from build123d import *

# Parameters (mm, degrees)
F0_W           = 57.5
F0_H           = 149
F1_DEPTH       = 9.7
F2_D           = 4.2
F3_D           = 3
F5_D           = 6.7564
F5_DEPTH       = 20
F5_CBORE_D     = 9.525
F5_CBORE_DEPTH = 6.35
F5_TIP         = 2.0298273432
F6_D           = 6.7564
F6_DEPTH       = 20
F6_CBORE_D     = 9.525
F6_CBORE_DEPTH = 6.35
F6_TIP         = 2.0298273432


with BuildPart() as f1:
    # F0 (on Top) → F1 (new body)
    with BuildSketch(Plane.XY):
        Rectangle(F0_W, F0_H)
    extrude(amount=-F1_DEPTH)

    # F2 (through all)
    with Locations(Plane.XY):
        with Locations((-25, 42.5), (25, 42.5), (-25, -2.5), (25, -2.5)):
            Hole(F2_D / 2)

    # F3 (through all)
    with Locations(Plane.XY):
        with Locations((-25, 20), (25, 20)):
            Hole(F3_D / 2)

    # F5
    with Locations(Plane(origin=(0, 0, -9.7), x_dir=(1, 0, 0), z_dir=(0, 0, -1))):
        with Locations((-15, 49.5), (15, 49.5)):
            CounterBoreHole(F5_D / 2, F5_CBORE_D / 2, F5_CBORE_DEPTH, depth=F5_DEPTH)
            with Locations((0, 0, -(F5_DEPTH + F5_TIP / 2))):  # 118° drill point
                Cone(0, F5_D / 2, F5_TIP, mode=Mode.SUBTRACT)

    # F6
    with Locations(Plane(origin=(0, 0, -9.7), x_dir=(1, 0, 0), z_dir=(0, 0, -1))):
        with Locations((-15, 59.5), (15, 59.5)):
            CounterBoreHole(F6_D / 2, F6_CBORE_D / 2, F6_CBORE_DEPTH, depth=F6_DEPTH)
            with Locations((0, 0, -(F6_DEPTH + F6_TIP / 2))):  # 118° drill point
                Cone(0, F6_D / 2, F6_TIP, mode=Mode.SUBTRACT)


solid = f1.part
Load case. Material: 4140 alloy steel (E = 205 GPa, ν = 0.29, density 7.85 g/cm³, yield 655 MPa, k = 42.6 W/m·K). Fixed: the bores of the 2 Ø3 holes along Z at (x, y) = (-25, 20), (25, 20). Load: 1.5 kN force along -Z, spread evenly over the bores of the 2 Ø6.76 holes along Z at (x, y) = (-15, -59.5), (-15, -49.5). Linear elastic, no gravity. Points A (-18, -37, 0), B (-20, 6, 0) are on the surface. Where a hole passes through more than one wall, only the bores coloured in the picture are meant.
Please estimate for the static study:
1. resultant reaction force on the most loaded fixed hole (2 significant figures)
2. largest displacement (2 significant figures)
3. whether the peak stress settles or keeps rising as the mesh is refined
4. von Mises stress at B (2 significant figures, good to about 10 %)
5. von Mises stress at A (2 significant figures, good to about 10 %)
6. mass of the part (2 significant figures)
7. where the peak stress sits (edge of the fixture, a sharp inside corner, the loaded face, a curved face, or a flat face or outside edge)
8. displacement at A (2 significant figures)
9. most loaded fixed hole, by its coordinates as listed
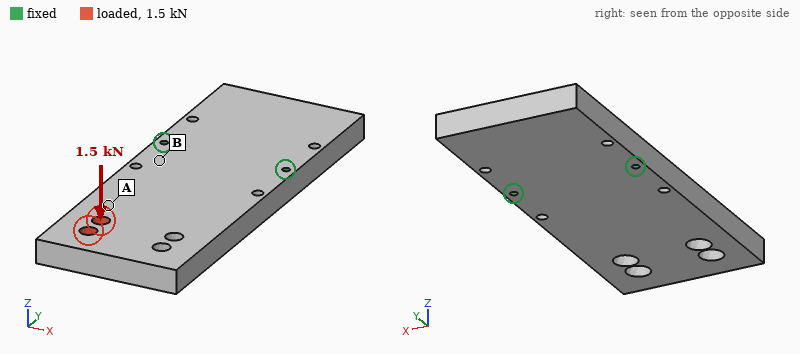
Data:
1.2 kN
0.47 mm
keeps rising
120 MPa
42 MPa
630 g
edge of the fixture
0.24 mm
(-25, 20)
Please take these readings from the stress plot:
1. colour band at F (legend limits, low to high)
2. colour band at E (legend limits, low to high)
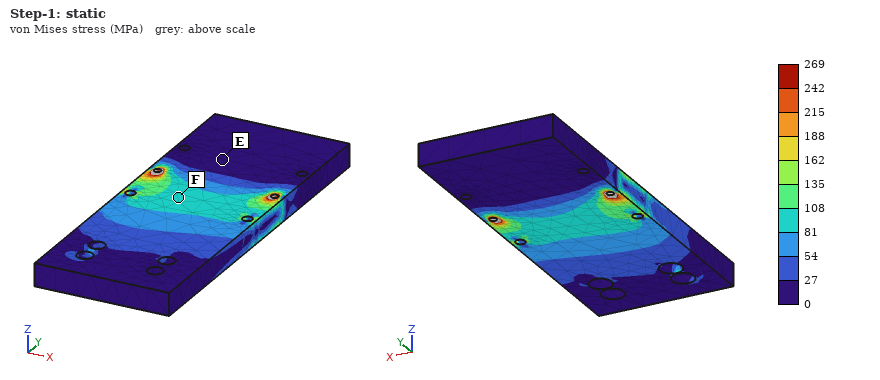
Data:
81 to 108 MPa
0 to 27 MPa
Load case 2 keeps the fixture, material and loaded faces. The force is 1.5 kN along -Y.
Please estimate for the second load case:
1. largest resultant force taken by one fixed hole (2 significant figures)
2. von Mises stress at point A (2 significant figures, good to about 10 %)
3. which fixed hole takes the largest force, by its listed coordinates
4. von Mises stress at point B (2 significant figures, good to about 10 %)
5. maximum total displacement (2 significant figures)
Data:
1.2 kN
12 MPa
(-25, 20)
12 MPa
30 µm
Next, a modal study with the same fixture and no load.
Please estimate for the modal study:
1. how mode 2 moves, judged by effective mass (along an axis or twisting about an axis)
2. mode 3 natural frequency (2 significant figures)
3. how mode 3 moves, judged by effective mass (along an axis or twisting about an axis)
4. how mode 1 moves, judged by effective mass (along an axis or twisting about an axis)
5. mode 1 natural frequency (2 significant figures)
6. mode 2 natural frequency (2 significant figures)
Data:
along Z
3000 Hz
twisting about Y
along Z
780 Hz
2200 Hz
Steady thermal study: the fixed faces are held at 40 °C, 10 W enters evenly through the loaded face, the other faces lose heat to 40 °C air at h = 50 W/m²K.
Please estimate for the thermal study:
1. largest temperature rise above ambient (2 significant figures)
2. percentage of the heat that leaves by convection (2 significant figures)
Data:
27 K
71 %
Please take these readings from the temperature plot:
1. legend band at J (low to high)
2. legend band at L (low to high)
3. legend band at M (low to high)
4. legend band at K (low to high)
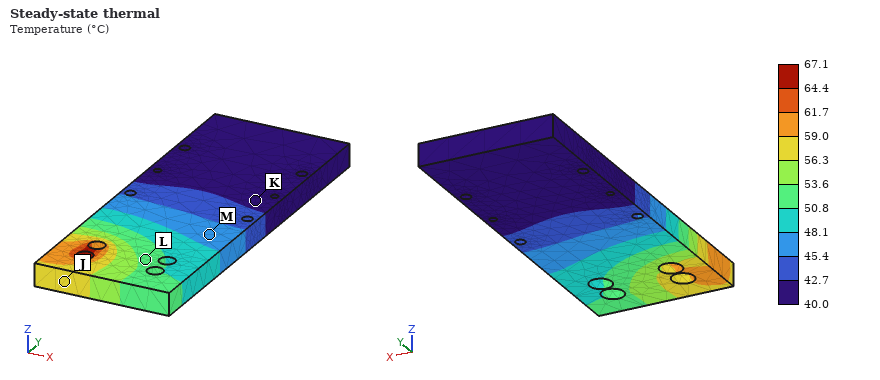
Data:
56.3 to 59.0 °C
50.8 to 53.6 °C
45.4 to 48.1 °C
40.0 to 42.7 °C
